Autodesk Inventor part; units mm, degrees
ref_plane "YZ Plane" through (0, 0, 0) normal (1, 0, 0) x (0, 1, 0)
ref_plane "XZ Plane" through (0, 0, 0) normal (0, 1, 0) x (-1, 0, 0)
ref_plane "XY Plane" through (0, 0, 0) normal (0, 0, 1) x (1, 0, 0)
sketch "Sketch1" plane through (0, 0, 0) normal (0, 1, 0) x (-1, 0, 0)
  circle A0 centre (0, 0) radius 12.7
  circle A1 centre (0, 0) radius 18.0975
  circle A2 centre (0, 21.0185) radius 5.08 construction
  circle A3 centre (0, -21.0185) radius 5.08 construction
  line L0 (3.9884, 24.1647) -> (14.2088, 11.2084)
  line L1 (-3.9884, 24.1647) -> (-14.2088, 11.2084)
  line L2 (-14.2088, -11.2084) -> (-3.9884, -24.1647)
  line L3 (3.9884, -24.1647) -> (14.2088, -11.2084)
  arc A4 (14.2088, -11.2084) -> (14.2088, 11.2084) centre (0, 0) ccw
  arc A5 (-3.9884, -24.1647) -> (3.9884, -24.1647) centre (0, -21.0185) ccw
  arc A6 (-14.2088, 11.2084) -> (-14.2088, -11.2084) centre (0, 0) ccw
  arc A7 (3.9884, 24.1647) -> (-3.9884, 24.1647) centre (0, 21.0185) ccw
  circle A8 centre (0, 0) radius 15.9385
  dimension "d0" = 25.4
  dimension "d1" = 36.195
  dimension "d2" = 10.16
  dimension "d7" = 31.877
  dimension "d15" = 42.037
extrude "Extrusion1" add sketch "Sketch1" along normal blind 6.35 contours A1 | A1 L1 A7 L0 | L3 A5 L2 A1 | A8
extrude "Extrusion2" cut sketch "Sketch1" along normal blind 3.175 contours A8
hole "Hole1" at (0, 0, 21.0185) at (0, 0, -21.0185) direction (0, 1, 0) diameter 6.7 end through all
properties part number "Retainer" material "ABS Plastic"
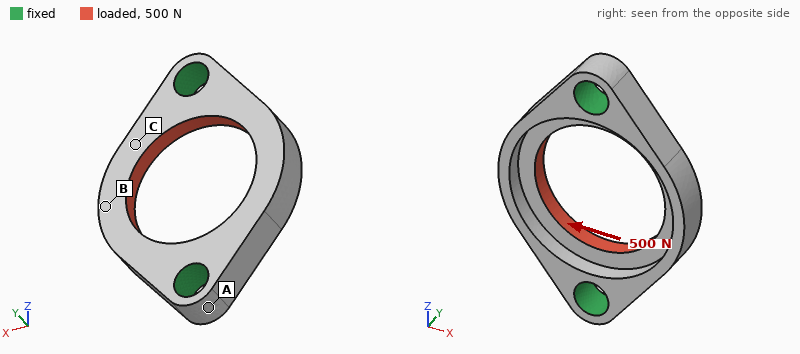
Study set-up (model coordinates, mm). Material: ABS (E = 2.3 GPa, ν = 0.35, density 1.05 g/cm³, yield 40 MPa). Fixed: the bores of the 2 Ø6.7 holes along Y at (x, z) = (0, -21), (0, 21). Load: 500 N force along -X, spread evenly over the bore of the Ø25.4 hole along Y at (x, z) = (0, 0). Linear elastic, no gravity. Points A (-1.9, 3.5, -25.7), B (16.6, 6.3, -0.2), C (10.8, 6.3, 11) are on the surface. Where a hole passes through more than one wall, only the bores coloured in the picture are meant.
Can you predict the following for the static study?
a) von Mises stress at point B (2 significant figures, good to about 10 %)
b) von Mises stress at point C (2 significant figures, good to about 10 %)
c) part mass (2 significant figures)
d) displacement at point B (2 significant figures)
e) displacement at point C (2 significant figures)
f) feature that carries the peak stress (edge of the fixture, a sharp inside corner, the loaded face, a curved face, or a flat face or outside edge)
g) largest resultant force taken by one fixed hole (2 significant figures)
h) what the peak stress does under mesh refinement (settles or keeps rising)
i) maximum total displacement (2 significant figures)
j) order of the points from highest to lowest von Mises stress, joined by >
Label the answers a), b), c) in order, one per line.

a) 5.3 MPa
b) 6.6 MPa
c) 3.5 g
d) 0.11 mm
e) 0.058 mm
f) edge of the fixture
g) 250 N
h) keeps rising
i) 0.12 mm
j) C > B > A
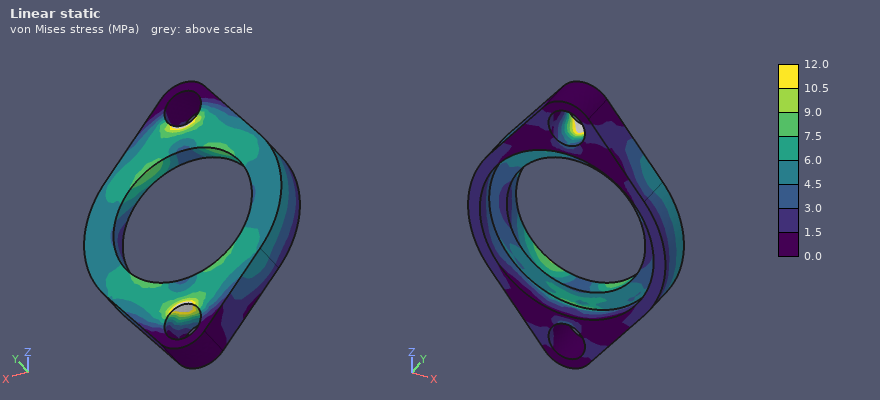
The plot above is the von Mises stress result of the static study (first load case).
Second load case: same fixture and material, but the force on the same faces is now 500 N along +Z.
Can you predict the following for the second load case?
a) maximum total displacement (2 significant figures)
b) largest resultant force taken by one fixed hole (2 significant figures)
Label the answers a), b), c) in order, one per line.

a) 78 µm
b) 250 N
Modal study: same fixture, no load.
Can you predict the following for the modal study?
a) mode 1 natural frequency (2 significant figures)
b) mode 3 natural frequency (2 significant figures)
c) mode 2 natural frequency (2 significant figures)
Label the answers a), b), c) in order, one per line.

a) 3400 Hz
b) 7000 Hz
c) 3600 Hz
